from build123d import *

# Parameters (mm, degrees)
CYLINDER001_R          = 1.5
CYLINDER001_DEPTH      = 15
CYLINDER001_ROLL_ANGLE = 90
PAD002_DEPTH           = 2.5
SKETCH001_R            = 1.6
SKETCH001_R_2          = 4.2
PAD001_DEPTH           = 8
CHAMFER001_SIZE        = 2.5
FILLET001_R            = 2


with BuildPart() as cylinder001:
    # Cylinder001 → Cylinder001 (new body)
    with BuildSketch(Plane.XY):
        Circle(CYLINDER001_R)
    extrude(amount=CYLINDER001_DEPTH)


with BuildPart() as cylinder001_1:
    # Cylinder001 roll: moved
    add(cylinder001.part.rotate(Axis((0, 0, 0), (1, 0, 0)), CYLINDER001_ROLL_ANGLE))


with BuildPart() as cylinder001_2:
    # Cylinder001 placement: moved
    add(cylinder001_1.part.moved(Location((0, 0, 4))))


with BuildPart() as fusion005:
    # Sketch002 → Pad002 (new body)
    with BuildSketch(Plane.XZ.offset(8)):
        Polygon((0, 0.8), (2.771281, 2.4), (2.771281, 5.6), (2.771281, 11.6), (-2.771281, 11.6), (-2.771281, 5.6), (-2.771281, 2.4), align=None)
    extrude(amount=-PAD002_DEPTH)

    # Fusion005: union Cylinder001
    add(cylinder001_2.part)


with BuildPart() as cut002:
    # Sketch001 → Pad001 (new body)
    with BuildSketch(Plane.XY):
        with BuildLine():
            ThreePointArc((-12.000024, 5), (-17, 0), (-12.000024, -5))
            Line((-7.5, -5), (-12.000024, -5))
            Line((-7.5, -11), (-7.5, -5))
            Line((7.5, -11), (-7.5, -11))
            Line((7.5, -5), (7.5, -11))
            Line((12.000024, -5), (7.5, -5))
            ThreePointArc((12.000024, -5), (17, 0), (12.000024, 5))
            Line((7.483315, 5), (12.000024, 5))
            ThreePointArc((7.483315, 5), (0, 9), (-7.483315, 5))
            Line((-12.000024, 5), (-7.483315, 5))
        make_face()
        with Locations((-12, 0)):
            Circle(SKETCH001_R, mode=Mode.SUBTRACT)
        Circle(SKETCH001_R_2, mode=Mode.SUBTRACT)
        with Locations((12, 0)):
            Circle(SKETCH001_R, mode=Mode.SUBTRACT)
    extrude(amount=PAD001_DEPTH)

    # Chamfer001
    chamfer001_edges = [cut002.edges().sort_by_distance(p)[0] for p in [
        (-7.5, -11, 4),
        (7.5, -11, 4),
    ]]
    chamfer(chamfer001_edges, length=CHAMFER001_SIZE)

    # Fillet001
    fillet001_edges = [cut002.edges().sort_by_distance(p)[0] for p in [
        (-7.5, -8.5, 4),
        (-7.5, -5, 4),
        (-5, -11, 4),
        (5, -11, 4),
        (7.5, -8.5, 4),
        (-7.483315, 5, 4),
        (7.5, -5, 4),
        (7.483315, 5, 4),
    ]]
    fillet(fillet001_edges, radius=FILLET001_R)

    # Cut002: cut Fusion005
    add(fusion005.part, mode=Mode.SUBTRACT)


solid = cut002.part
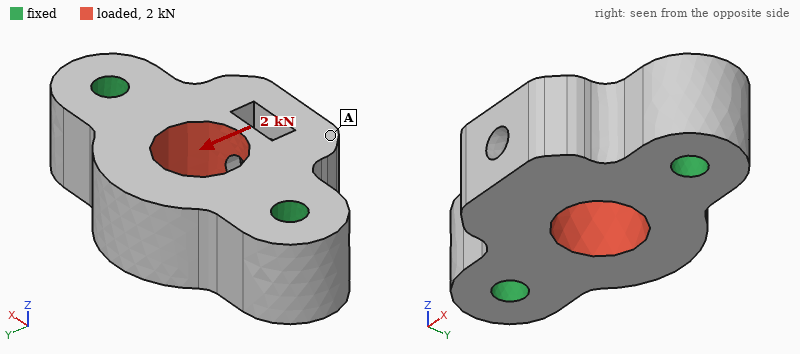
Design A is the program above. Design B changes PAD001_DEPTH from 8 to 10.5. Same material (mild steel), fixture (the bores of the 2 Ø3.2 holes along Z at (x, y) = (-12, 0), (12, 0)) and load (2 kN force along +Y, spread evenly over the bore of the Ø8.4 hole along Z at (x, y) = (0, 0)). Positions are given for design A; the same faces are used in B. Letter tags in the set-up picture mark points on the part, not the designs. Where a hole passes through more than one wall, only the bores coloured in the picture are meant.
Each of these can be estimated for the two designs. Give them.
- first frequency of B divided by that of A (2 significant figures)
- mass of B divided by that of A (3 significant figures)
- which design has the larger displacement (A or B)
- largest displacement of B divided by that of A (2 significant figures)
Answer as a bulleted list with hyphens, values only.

- 1.1
- 1.31
- A
- 0.78
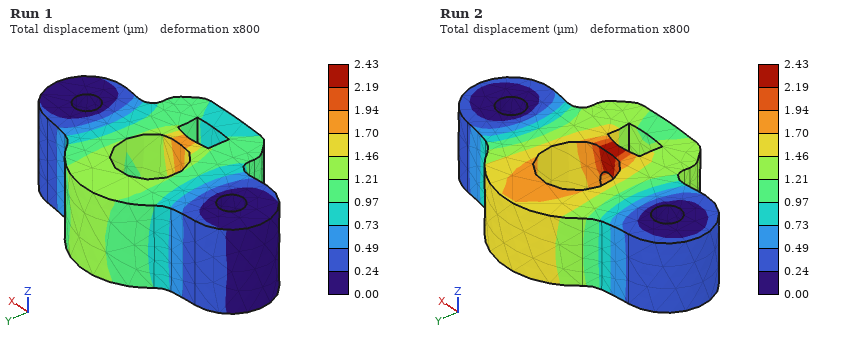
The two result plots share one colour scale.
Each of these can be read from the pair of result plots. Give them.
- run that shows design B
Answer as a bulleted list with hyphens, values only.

- Run 1
